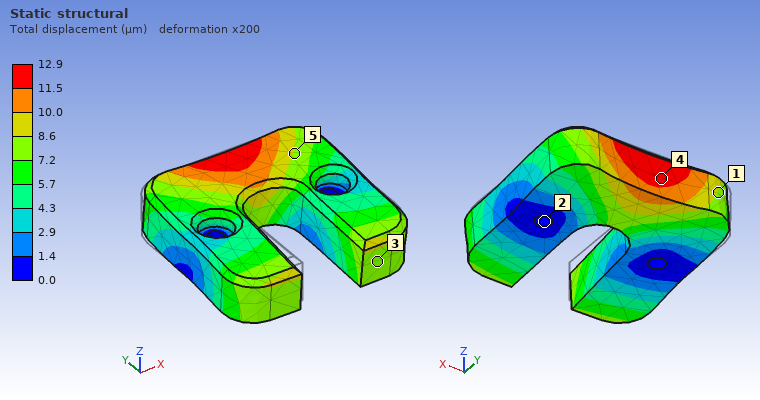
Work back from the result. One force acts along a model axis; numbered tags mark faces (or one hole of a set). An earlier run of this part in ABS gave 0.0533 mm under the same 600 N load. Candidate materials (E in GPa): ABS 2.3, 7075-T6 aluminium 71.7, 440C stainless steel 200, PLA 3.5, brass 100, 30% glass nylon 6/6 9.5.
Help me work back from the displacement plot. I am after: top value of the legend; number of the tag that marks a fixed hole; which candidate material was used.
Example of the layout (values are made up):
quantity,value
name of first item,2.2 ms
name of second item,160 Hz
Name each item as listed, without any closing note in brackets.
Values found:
quantity,value
top value of the legend,12.9 µm
number of the tag that marks a fixed hole,2
which candidate material was used,30% glass nylon 6/6
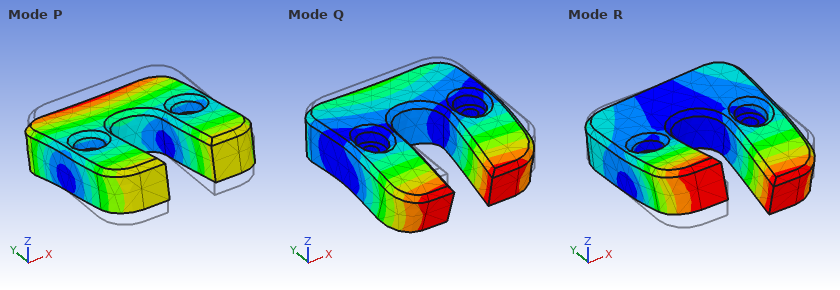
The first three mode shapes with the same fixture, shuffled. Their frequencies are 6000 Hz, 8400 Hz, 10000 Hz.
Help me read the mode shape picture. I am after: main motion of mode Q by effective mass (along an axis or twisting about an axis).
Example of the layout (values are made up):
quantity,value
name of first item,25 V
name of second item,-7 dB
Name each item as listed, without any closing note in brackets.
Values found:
quantity,value
main motion of mode Q by effective mass,along Z
